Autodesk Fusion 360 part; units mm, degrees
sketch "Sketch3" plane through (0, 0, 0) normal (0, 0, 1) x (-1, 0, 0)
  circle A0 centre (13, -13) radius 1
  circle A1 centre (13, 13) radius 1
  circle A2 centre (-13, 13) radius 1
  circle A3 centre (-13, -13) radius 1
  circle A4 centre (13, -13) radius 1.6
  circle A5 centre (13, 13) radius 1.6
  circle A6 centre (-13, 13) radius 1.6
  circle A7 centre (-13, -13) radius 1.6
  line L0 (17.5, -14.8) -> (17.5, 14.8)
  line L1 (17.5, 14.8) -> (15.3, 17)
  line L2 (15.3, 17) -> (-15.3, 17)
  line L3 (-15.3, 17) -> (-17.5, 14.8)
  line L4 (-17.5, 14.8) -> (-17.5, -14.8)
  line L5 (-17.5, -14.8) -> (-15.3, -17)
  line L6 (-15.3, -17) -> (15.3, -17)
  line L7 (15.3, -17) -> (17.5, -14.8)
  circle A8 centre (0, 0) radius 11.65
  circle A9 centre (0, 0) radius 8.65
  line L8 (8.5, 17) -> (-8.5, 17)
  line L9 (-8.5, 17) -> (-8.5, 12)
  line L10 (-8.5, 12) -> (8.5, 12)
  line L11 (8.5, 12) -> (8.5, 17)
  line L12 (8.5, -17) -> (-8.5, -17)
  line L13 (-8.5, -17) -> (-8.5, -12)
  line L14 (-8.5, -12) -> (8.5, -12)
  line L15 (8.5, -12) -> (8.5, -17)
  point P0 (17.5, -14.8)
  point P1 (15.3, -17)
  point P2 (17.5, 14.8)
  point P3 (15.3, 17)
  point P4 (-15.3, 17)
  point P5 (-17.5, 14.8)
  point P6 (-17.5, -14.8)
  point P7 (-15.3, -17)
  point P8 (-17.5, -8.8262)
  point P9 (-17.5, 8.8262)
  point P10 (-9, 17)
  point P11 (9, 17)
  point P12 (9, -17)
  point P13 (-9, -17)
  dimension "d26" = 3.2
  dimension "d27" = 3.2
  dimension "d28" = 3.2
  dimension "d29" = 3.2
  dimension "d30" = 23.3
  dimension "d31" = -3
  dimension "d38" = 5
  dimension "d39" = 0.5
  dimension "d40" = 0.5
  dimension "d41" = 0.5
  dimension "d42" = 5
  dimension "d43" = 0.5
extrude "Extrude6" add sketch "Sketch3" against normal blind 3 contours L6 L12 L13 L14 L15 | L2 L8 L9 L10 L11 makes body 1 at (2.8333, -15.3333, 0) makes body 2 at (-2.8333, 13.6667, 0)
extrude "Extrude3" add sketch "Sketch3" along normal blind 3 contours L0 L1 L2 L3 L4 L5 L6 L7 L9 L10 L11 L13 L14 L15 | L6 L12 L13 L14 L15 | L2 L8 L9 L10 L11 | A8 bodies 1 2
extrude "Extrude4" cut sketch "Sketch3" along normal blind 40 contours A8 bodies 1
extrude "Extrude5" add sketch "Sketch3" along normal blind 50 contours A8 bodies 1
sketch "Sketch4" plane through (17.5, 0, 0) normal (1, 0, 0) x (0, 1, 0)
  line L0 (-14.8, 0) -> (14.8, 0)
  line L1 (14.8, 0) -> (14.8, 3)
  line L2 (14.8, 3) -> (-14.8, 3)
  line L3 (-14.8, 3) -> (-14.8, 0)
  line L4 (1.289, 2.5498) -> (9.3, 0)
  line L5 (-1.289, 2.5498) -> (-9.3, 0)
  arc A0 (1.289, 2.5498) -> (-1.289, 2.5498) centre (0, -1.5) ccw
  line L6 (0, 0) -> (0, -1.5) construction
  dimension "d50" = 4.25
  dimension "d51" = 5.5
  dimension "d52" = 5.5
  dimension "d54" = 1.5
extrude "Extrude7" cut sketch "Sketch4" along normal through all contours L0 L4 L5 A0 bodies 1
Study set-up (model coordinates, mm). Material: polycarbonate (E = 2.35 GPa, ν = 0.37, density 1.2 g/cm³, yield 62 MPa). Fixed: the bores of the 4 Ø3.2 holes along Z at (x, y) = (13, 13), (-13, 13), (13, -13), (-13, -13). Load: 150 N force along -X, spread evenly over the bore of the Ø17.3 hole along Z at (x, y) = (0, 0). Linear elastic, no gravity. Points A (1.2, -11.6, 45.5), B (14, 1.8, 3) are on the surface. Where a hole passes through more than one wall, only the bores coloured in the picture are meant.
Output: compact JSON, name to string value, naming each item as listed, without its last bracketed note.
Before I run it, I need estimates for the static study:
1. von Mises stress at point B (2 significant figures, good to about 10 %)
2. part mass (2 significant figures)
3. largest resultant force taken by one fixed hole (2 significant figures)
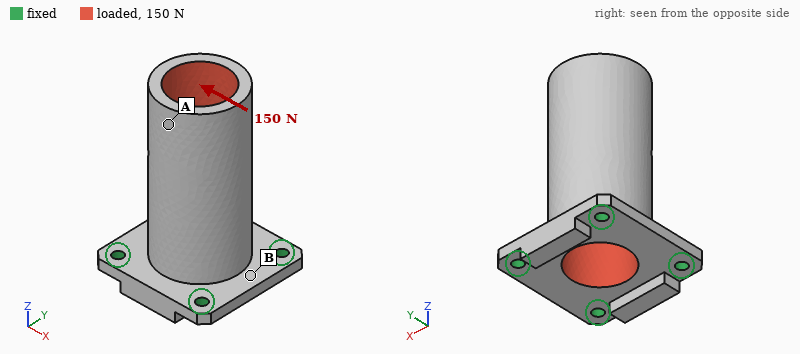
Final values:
{"von Mises stress at point B": "5.3 MPa", "part mass": "15 g", "largest resultant force taken by one fixed hole": "90 N"}
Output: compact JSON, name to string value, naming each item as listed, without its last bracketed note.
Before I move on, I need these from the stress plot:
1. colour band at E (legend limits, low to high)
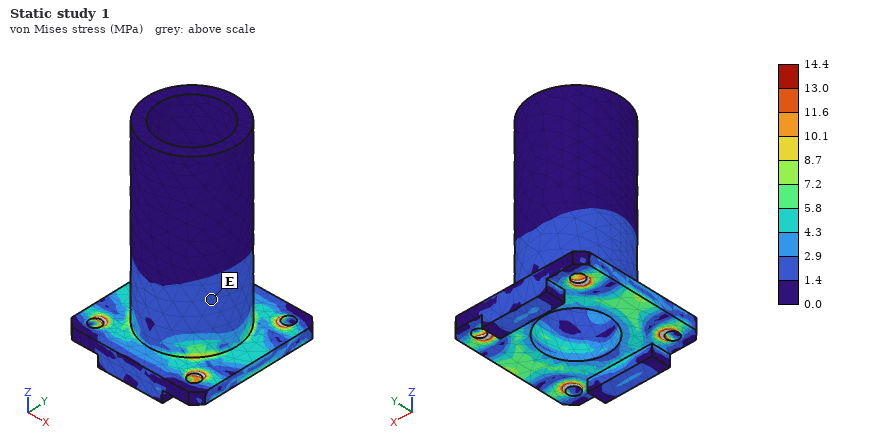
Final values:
{"colour band at E": "1.4 to 2.9 MPa"}
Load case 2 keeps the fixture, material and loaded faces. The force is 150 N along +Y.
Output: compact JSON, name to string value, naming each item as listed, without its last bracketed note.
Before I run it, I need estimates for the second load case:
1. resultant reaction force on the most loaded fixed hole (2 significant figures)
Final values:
{"resultant reaction force on the most loaded fixed hole": "84 N"}
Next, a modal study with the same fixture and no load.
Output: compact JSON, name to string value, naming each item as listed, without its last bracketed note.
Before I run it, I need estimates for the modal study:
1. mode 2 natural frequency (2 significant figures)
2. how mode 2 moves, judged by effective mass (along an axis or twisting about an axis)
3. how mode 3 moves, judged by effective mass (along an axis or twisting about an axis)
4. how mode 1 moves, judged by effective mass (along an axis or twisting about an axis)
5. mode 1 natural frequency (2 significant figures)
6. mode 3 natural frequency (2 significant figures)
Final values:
{"mode 2 natural frequency": "1100 Hz", "how mode 2 moves, judged by effective mass": "along Y", "how mode 3 moves, judged by effective mass": "along Z", "how mode 1 moves, judged by effective mass": "along X", "mode 1 natural frequency": "1000 Hz", "mode 3 natural frequency": "2900 Hz"}
